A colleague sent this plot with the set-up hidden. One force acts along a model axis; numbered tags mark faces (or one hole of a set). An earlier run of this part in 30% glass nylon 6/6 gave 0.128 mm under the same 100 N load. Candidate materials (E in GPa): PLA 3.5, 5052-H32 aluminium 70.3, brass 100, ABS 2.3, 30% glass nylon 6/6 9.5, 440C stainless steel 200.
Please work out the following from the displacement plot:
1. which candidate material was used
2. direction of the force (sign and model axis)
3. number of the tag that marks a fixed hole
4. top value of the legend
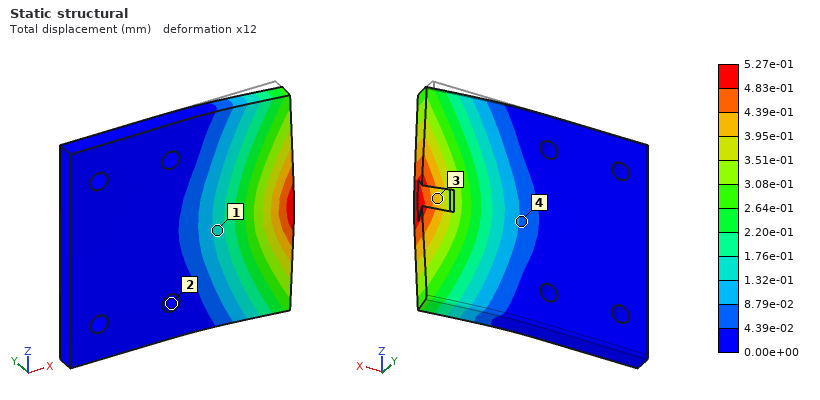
ABS
-Y
2
5.27e-01 mm
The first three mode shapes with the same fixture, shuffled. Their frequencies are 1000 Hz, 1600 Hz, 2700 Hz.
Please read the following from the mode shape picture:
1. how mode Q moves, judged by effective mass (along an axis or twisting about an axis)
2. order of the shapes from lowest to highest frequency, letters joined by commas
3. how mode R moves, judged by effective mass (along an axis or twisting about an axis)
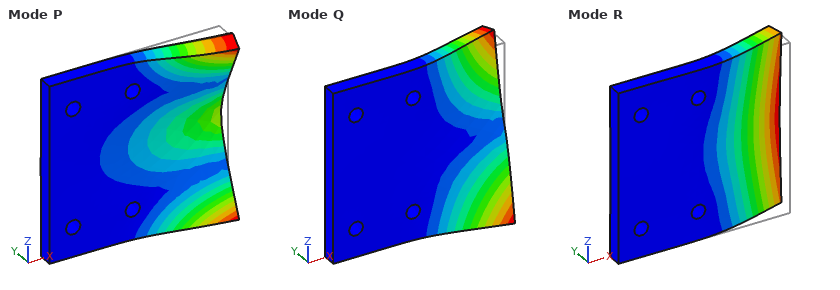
twisting about X
R, Q, P
along Y
